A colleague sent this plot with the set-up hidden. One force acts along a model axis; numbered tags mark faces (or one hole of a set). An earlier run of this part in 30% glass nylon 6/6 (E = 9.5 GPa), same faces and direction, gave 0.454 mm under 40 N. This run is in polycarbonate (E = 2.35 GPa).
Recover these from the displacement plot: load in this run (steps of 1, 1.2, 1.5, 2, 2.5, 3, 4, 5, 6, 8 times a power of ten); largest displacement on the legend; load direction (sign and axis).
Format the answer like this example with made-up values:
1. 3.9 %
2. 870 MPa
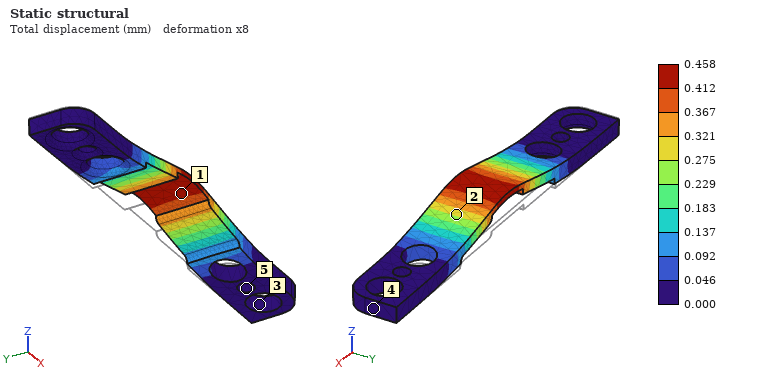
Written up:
1. 10 N
2. 0.458 mm
3. +Z
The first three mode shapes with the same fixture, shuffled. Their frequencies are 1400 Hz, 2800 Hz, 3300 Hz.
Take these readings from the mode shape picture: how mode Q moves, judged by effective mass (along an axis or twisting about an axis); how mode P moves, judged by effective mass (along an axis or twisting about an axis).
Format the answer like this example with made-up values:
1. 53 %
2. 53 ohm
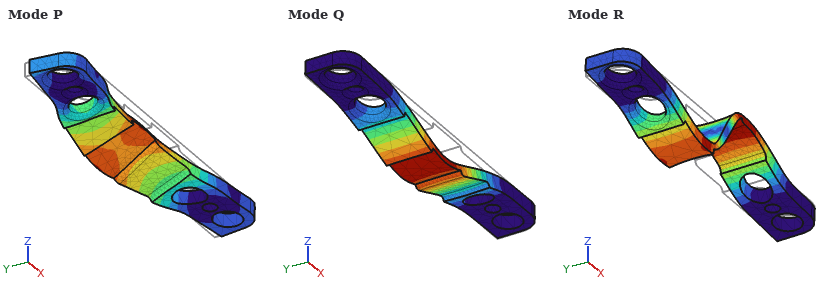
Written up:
1. along Z
2. along Y
